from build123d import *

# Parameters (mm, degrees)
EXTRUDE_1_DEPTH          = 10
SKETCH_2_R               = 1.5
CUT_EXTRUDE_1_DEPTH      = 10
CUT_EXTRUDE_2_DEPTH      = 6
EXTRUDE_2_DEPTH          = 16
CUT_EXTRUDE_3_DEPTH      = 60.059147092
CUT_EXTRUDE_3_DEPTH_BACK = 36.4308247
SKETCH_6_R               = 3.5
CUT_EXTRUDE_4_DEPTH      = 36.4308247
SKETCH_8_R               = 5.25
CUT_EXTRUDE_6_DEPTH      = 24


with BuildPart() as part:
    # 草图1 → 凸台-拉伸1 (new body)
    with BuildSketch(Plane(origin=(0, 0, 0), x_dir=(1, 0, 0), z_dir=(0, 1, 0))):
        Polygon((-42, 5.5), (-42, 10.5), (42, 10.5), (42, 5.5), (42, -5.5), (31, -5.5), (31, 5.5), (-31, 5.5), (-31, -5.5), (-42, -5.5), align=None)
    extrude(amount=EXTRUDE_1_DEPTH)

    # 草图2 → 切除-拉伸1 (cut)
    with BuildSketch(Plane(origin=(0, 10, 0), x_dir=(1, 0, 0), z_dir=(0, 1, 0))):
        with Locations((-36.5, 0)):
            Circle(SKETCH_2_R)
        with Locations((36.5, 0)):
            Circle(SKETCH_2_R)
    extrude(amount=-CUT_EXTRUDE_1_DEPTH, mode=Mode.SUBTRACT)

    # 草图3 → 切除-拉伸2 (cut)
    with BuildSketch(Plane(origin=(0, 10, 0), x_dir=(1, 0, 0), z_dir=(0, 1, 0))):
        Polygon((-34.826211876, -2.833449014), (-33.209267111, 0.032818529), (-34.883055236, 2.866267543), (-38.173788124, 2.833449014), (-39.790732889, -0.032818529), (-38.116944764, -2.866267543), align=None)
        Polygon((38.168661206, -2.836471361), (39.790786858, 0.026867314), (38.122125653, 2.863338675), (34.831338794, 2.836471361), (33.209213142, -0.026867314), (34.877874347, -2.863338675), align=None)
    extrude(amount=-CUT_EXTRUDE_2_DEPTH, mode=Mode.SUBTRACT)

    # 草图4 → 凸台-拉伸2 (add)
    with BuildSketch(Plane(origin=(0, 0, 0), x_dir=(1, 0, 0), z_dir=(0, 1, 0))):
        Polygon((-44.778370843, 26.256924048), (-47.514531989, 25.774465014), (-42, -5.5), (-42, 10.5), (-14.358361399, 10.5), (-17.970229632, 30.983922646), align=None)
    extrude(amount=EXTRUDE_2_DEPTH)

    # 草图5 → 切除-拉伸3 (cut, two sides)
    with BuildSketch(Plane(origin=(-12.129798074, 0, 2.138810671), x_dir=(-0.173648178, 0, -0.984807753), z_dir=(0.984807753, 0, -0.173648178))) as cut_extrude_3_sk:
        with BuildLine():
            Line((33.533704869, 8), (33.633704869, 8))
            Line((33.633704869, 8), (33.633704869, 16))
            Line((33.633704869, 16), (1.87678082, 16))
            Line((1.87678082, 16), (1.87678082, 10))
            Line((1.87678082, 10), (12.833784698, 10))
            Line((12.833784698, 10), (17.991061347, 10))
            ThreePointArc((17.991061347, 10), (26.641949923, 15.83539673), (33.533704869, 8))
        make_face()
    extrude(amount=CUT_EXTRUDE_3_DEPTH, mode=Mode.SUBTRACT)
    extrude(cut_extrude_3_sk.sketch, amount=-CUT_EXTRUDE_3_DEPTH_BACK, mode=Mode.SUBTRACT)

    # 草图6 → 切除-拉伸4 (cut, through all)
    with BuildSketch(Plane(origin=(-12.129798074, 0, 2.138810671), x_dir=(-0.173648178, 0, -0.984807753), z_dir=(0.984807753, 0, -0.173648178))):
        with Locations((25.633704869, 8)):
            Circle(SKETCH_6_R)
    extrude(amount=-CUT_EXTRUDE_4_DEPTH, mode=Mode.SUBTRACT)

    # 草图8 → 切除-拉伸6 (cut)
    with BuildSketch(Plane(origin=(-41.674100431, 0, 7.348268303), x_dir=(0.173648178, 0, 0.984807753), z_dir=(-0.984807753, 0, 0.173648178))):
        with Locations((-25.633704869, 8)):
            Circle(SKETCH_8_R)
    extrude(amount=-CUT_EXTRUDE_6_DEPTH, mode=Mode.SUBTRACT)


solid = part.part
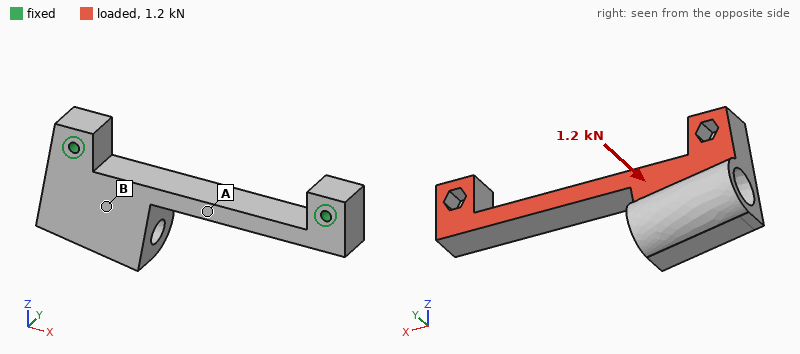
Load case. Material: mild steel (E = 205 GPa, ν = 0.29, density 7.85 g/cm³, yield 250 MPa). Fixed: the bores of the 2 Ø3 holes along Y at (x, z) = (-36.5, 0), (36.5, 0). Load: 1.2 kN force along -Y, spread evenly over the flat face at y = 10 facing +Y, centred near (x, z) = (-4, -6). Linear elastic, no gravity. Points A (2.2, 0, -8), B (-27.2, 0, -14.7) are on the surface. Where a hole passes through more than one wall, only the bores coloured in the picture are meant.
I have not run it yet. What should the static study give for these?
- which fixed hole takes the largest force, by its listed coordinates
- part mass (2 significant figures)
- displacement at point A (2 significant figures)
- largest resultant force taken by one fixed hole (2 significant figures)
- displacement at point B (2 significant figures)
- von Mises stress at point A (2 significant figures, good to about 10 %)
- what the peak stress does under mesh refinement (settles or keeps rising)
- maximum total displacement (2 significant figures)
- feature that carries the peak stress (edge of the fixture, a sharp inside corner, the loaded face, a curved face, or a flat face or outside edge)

(-36.5, 0)
91 g
20 µm
680 N
14 µm
32 MPa
keeps rising
29 µm
edge of the fixture
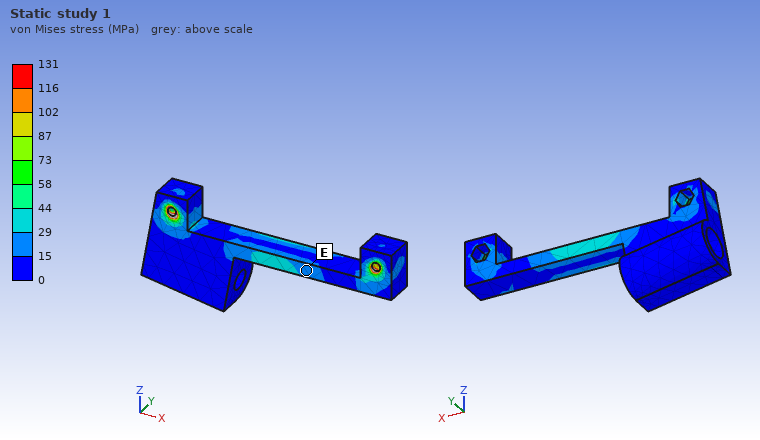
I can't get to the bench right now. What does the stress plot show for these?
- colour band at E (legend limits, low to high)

15 to 29 MPa
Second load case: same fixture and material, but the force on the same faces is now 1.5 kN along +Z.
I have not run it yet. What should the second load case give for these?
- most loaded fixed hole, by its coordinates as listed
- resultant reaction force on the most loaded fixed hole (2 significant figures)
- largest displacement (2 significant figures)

(-36.5, 0)
1000 N
45 µm
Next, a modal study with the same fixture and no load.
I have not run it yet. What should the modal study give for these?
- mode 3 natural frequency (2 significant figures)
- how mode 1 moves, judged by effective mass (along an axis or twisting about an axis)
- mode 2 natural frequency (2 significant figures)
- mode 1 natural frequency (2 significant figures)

5900 Hz
along Y
4000 Hz
3000 Hz
